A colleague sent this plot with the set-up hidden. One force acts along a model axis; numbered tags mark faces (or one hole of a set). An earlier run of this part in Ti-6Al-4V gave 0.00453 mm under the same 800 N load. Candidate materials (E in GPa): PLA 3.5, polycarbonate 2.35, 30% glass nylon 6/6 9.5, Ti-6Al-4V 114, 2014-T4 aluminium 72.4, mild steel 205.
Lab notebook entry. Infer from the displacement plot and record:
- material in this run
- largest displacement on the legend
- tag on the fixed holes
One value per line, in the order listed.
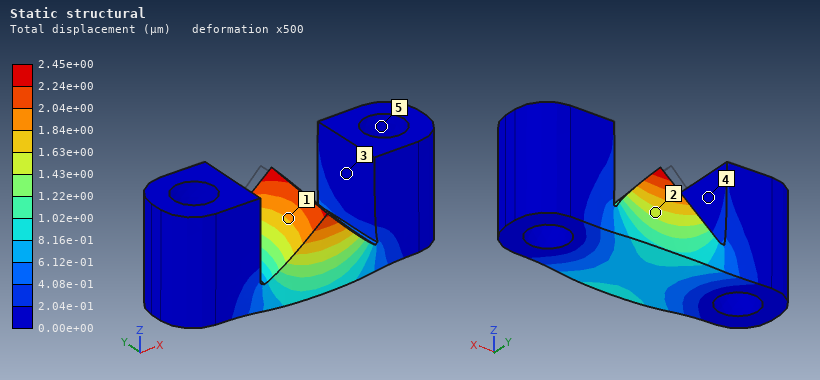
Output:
mild steel
2.45e+00 µm
5
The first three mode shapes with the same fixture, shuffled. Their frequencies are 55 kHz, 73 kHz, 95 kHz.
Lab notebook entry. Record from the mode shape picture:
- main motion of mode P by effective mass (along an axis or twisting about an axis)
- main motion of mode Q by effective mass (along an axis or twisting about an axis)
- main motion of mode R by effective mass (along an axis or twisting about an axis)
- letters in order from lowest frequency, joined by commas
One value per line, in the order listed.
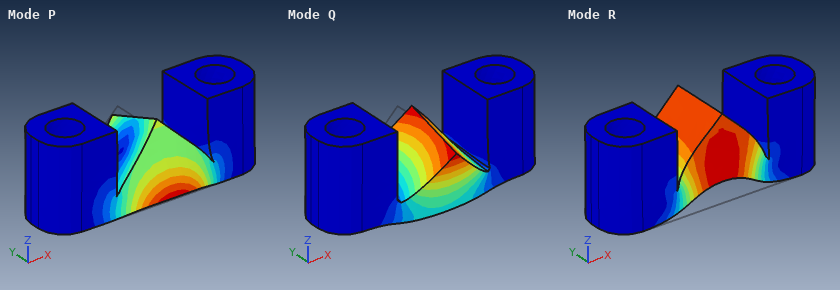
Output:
along Y
along Y
along Z
Q, R, P
